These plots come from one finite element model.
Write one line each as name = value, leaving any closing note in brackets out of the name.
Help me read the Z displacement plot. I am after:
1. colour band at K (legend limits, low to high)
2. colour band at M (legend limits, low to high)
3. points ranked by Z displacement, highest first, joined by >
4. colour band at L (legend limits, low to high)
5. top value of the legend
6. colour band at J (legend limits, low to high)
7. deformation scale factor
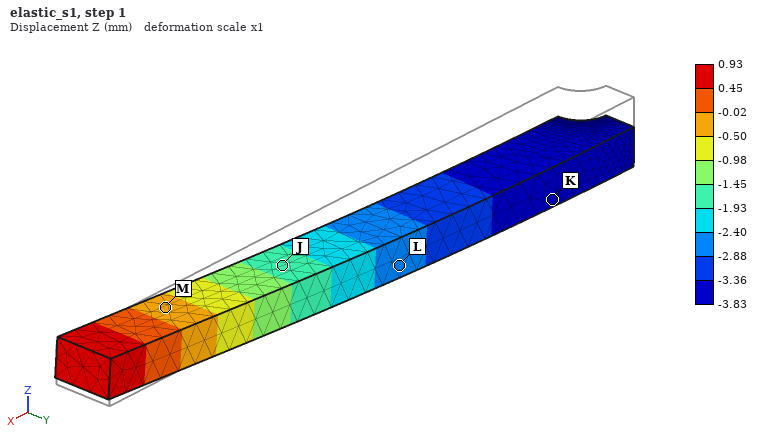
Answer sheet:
colour band at K = -3.83 to -3.36 mm
colour band at M = -0.50 to -0.02 mm
points ranked by Z displacement, highest first, joined by > = M > J > L > K
colour band at L = -2.88 to -2.40 mm
top value of the legend = 0.93 mm
colour band at J = -1.93 to -1.45 mm
deformation scale factor = 1
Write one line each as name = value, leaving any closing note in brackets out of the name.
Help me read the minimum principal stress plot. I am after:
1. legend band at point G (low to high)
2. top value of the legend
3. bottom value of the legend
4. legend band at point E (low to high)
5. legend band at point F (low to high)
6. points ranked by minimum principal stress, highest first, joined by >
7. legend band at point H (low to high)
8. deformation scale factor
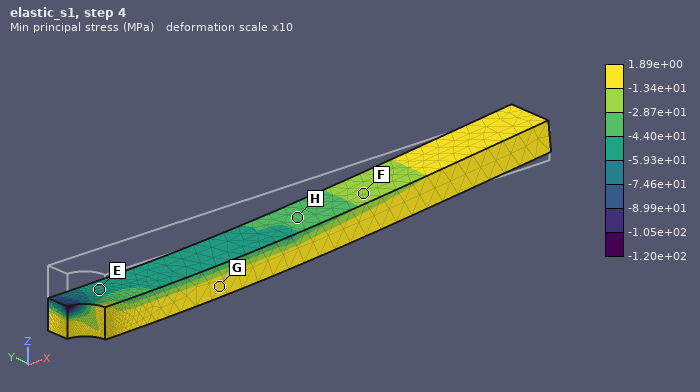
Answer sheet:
legend band at point G = -1.34e+01 to 1.89e+00 MPa
top value of the legend = 1.89e+00 MPa
bottom value of the legend = -1.20e+02 MPa
legend band at point E = -5.93e+01 to -4.40e+01 MPa
legend band at point F = -2.87e+01 to -1.34e+01 MPa
points ranked by minimum principal stress, highest first, joined by > = G > F > H > E
legend band at point H = -4.40e+01 to -2.87e+01 MPa
deformation scale factor = 10
